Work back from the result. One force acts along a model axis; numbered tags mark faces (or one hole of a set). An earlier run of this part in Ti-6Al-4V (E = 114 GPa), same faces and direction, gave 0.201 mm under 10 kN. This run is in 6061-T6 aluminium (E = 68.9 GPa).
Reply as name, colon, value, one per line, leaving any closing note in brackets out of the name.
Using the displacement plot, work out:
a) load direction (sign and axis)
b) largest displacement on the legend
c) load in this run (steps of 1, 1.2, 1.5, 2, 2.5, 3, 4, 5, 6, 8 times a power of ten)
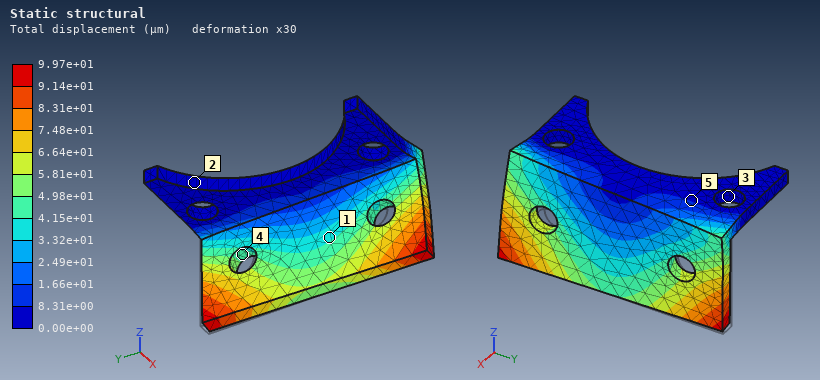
load direction: -Y
largest displacement on the legend: 9.97e+01 µm
load in this run: 3 kN
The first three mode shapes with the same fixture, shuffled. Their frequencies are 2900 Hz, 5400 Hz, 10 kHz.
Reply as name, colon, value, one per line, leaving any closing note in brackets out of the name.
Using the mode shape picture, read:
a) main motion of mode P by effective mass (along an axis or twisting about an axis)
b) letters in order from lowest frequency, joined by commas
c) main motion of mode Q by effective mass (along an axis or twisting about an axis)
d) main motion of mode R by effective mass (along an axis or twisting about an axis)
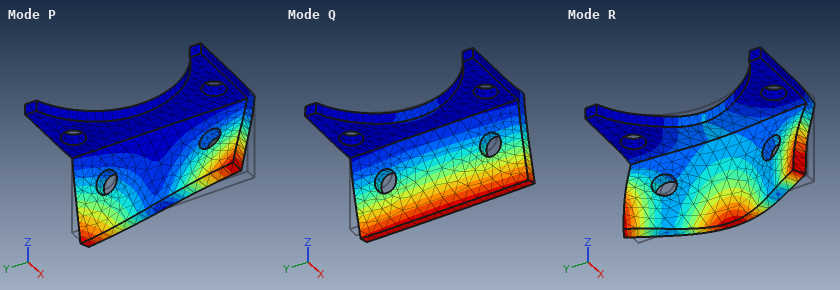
main motion of mode P by effective mass: twisting about Z
letters in order from lowest frequency, joined by commas: Q, P, R
main motion of mode Q by effective mass: along X
main motion of mode R by effective mass: along Z
